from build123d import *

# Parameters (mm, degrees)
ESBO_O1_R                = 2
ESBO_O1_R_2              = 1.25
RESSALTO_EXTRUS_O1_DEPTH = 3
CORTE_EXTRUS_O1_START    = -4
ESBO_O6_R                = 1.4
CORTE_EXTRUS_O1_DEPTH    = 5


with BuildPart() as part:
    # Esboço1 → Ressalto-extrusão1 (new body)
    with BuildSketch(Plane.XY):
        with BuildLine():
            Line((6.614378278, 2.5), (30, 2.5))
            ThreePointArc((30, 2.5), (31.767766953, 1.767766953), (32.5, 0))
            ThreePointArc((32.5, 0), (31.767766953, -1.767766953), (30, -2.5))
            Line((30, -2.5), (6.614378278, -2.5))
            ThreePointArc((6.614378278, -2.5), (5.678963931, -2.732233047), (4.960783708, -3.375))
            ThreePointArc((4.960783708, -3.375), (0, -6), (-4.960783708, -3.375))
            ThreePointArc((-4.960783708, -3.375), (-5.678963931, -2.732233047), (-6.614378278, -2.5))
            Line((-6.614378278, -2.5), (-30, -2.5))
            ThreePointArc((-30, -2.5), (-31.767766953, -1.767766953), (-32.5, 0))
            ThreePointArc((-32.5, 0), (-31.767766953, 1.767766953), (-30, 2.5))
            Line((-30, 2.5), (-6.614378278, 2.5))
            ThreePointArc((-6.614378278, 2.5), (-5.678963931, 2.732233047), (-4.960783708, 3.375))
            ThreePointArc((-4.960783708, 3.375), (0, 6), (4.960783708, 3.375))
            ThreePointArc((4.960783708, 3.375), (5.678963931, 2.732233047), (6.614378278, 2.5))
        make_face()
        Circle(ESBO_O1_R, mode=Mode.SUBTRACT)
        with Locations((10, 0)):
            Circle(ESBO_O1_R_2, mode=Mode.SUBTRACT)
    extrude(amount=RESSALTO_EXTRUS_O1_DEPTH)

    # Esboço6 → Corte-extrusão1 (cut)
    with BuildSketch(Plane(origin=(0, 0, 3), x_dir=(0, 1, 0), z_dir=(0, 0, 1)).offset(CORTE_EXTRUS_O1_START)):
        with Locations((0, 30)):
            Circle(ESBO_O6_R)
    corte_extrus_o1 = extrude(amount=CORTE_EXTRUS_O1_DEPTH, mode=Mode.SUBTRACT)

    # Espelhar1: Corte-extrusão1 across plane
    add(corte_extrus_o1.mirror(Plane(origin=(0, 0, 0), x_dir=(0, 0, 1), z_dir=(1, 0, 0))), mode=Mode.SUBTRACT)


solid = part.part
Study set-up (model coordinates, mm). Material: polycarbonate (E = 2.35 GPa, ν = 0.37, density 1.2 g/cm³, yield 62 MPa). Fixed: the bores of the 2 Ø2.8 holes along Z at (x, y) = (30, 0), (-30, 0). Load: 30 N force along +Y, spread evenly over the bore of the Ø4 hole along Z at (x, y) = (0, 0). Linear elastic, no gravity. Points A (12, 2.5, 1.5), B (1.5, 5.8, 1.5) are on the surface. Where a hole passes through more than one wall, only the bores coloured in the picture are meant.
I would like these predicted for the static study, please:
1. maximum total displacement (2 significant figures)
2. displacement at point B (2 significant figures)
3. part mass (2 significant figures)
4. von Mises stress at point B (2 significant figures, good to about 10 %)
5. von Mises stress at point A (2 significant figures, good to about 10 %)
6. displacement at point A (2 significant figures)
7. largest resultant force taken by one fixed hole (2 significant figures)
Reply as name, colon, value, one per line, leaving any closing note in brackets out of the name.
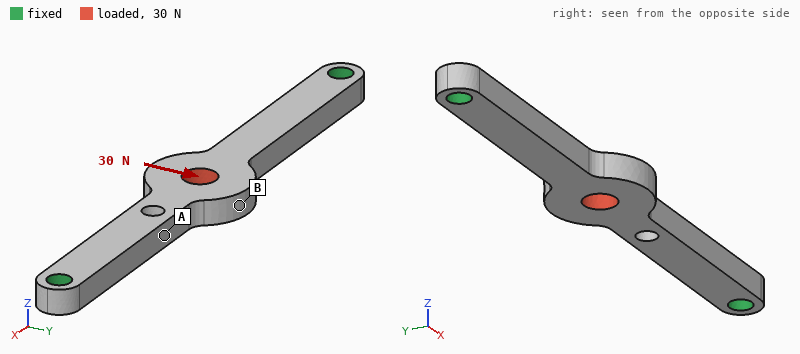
maximum total displacement: 0.35 mm
displacement at point B: 0.34 mm
part mass: 1.2 g
von Mises stress at point B: 1.7 MPa
von Mises stress at point A: 4.3 MPa
displacement at point A: 0.26 mm
largest resultant force taken by one fixed hole: 15 N
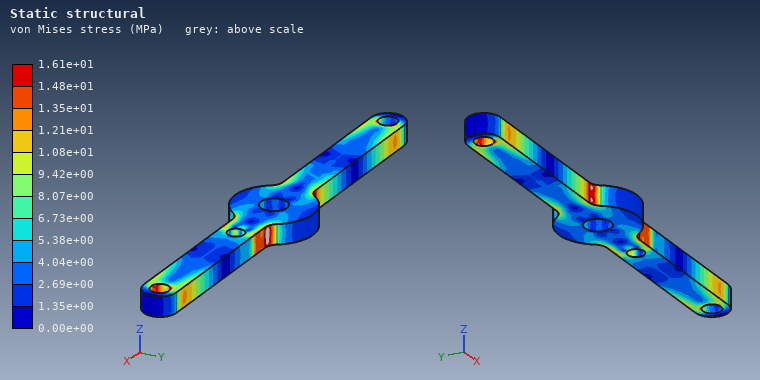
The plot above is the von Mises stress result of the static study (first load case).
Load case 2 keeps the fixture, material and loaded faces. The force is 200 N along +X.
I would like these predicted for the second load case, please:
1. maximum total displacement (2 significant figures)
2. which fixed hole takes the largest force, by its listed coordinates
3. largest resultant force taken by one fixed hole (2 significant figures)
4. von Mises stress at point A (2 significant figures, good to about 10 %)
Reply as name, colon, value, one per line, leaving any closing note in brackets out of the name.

maximum total displacement: 85 µm
which fixed hole takes the largest force, by its listed coordinates: (-30, 0)
largest resultant force taken by one fixed hole: 110 N
von Mises stress at point A: 11 MPa
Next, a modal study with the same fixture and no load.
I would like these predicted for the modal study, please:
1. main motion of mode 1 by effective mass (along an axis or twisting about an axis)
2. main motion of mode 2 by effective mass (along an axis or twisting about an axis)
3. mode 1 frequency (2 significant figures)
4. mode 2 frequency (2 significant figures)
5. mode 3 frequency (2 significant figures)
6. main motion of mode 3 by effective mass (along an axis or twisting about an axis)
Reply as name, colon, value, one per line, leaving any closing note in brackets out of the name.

main motion of mode 1 by effective mass: along Z
main motion of mode 2 by effective mass: along Y
mode 1 frequency: 1100 Hz
mode 2 frequency: 1900 Hz
mode 3 frequency: 3200 Hz
main motion of mode 3 by effective mass: twisting about X
